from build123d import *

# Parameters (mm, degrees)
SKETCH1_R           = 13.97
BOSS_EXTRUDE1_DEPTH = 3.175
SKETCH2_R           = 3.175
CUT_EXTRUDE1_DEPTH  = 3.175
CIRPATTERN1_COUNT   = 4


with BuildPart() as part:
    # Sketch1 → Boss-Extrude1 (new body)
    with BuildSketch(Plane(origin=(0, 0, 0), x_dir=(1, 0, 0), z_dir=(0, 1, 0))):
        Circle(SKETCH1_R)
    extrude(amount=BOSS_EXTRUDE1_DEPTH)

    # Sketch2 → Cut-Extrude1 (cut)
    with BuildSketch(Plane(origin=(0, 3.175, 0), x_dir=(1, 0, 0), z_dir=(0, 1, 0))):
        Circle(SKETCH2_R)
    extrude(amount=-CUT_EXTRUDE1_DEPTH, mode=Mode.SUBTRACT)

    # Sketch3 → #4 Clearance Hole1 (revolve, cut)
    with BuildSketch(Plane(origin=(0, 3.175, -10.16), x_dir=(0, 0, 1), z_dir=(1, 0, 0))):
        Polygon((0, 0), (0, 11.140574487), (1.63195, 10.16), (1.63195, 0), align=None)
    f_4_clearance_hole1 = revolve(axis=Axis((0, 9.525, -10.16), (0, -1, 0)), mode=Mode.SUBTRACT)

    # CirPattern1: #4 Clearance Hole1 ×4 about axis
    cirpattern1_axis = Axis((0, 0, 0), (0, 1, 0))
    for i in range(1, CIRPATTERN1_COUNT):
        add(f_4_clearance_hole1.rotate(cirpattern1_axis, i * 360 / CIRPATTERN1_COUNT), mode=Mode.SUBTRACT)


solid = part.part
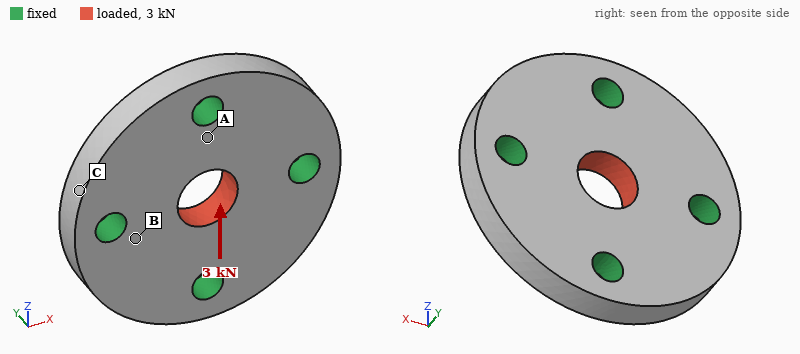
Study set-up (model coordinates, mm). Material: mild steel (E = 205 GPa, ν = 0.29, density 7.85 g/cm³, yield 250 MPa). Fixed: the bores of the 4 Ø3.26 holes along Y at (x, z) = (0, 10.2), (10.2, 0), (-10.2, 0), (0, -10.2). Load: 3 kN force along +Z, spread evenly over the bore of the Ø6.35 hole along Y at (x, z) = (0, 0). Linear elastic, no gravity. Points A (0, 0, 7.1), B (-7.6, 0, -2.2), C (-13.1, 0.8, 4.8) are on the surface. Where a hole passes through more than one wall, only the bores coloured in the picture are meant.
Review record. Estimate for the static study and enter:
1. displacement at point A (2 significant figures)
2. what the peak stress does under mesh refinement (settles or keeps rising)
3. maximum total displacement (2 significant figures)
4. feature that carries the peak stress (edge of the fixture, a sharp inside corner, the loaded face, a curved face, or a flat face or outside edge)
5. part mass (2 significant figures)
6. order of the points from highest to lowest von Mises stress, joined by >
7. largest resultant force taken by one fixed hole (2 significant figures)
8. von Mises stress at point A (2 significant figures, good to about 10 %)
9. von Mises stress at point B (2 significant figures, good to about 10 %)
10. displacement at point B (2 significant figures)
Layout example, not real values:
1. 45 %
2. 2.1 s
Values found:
1. 0.43 µm
2. keeps rising
3. 1.8 µm
4. edge of the fixture
5. 14 g
6. A > B > C
7. 980 N
8. 62 MPa
9. 18 MPa
10. 0.43 µm
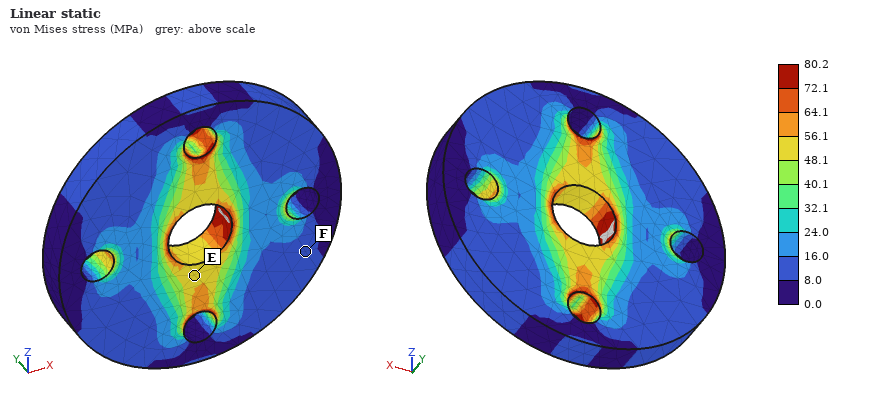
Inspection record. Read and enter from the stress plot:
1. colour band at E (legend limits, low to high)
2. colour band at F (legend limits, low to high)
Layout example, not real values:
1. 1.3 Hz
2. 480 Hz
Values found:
1. 48.1 to 56.1 MPa
2. 8.0 to 16.0 MPa
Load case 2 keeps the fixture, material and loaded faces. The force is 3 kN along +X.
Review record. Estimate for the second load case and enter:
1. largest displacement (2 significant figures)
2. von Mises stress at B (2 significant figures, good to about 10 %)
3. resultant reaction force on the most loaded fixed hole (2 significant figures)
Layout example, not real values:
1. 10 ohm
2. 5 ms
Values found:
1. 1.8 µm
2. 35 MPa
3. 980 N
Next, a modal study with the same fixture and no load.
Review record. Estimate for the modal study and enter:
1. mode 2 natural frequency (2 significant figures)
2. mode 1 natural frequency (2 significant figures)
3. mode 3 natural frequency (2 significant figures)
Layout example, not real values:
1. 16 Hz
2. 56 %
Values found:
1. 54 kHz
2. 52 kHz
3. 54 kHz
